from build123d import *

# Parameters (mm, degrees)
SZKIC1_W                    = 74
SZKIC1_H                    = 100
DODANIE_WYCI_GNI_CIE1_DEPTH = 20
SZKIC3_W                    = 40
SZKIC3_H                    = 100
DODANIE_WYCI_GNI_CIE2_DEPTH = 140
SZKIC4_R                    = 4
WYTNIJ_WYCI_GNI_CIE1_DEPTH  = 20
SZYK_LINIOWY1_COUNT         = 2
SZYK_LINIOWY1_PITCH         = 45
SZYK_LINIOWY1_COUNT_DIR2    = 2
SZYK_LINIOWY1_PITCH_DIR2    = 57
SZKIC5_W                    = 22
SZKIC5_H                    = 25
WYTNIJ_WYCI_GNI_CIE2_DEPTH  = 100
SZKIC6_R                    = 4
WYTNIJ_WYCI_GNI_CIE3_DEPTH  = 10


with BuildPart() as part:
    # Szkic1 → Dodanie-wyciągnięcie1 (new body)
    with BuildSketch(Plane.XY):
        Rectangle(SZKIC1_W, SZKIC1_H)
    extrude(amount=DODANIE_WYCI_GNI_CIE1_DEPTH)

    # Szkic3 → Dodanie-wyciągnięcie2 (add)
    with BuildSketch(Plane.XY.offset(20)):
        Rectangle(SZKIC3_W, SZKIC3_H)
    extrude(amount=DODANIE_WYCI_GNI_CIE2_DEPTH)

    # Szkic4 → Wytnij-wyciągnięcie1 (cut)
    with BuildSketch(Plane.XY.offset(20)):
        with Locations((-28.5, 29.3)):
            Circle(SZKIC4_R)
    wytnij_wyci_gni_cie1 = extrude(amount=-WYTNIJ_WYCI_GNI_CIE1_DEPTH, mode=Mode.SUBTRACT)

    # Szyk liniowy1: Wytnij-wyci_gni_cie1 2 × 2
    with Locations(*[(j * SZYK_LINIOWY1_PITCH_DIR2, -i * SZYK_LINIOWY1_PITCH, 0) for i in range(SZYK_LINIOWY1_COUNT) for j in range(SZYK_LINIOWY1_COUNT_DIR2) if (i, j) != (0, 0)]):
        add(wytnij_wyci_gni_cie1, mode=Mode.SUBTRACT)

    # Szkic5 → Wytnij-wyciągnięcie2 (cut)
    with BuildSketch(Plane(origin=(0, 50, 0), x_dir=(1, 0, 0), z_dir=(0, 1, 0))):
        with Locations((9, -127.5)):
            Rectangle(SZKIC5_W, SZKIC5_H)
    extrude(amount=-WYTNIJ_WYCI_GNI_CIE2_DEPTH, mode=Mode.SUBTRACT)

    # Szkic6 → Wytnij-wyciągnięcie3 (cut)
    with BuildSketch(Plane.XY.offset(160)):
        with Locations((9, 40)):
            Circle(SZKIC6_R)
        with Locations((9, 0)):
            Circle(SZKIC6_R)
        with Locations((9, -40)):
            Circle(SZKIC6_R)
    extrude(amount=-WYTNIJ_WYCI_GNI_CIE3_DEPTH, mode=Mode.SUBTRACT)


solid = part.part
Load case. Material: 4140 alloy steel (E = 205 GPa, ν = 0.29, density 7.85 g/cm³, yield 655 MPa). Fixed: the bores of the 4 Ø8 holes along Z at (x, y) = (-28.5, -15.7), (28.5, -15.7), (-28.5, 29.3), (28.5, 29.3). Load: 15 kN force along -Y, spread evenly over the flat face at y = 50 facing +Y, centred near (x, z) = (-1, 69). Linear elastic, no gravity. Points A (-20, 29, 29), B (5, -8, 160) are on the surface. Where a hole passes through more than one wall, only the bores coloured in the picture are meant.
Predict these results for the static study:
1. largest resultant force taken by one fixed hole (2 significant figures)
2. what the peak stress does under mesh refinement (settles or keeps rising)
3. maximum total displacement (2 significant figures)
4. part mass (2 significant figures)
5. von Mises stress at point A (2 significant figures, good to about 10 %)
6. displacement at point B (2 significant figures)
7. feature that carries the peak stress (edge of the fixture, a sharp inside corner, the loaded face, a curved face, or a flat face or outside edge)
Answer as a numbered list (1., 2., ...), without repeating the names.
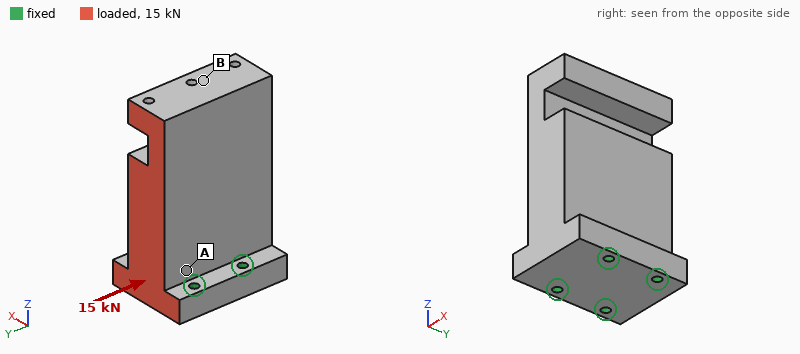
1. 8.6 kN
2. keeps rising
3. 34 µm
4. 5.1 kg
5. 15 MPa
6. 31 µm
7. edge of the fixture
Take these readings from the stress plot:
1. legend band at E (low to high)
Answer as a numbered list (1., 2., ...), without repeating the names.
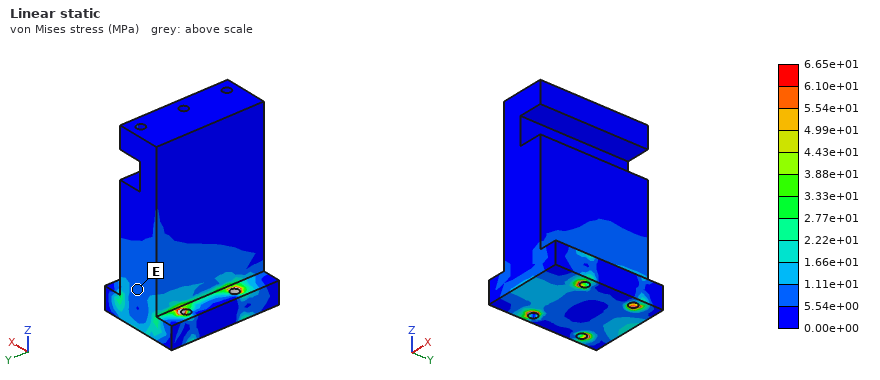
1. 5.54e+00 to 1.11e+01 MPa
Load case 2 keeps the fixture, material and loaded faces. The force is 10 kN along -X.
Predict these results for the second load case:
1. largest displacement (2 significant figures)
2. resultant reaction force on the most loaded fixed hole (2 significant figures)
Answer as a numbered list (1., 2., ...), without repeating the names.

1. 57 µm
2. 8.0 kN
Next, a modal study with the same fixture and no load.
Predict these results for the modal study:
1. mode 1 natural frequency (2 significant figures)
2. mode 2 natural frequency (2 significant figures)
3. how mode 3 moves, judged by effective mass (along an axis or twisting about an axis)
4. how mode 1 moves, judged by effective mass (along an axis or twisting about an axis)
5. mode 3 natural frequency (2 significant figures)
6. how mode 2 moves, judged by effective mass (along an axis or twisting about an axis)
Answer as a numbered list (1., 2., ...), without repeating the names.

1. 1400 Hz
2. 1800 Hz
3. twisting about Z
4. along X
5. 3500 Hz
6. along Y
